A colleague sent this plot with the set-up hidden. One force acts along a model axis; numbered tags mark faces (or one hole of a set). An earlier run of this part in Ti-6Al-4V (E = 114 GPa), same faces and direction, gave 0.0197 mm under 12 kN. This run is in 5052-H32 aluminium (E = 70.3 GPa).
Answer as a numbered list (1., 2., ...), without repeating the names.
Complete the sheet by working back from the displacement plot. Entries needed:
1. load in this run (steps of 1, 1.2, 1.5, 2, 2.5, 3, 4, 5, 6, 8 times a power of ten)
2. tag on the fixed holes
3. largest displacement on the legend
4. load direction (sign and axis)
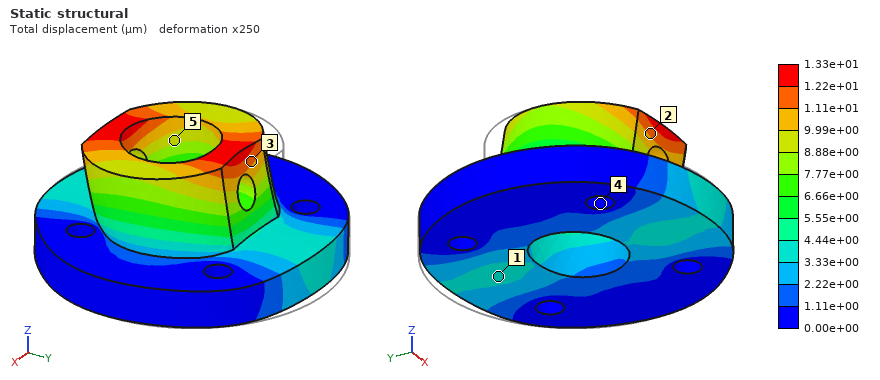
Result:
1. 5 kN
2. 4
3. 1.33e+01 µm
4. -Y
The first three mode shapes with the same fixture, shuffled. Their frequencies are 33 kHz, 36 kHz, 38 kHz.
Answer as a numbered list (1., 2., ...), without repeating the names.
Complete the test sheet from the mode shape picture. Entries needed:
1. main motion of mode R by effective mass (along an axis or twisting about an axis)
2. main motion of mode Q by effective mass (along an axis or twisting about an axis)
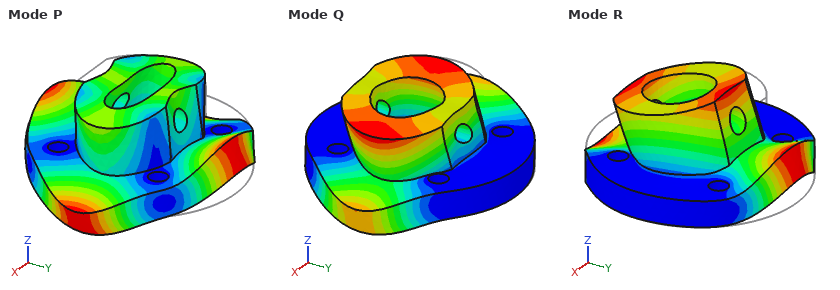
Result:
1. along Y
2. along X
